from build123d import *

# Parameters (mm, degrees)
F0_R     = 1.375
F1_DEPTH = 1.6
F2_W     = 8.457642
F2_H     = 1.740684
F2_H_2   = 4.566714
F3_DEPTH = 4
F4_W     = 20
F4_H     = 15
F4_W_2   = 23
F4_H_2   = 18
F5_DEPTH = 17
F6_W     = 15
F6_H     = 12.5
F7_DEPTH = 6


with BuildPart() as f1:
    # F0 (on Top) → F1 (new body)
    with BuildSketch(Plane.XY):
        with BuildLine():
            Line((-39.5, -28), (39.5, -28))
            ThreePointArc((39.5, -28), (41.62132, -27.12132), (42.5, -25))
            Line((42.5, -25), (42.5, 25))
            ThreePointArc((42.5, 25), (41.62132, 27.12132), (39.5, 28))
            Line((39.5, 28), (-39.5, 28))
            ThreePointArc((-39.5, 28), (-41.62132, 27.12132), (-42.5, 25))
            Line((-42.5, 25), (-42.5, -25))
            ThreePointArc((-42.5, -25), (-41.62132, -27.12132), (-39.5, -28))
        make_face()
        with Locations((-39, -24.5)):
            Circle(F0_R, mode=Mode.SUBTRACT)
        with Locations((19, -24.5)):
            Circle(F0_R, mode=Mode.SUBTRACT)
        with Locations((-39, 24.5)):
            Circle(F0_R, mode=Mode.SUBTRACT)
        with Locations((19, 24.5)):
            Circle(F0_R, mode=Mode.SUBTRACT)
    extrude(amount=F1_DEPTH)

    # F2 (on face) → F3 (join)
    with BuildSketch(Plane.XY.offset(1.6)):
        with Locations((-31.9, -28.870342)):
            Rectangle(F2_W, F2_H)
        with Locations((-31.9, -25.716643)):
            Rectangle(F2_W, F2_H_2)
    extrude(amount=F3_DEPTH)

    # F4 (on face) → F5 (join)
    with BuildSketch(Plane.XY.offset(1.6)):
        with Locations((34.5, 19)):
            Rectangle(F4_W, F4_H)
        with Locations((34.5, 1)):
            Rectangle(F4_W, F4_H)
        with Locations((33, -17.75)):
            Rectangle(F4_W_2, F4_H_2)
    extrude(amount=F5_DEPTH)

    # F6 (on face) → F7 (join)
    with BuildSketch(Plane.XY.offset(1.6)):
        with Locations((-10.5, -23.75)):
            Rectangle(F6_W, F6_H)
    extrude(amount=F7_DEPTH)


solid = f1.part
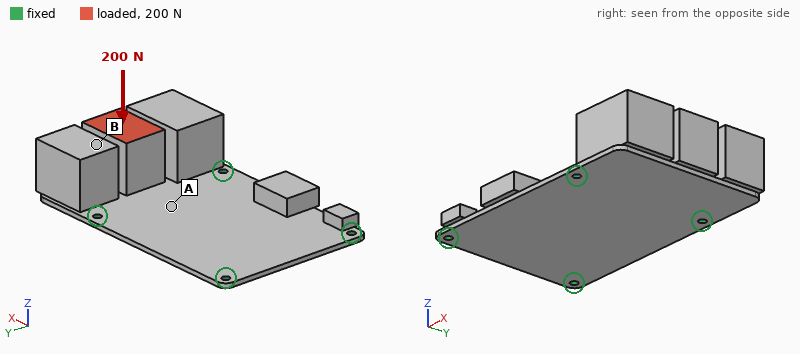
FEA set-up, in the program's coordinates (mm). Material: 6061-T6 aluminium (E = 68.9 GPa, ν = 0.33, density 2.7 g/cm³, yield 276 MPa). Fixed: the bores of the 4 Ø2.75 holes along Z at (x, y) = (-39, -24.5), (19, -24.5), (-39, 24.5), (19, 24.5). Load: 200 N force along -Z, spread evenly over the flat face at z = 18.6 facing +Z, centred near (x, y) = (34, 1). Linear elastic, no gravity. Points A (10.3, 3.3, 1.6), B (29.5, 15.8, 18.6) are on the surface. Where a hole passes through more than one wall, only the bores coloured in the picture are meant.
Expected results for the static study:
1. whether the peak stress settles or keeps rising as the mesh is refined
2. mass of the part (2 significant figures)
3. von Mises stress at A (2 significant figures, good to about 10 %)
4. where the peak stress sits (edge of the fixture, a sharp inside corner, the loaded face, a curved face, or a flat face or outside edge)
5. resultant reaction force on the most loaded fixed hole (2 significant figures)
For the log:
keeps rising
71 g
28 MPa
edge of the fixture
110 N
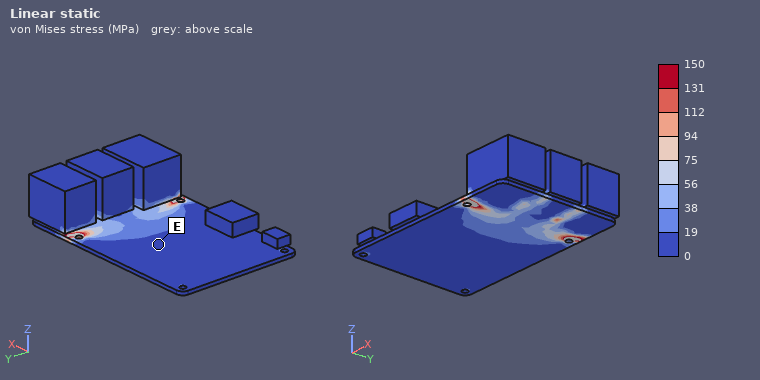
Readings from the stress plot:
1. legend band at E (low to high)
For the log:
0 to 19 MPa
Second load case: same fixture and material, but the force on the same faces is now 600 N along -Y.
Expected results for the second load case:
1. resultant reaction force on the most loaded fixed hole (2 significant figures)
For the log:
450 N
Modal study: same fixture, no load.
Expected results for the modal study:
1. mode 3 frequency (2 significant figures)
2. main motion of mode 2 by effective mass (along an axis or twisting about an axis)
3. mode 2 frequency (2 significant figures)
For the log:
2000 Hz
along Z
1600 Hz
